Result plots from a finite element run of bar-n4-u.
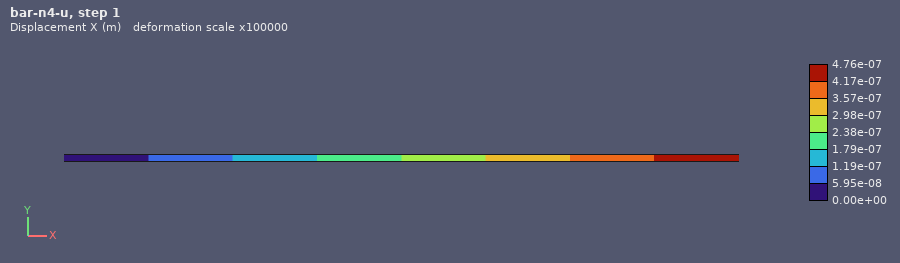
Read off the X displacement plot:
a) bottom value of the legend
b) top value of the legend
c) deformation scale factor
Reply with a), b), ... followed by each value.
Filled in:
a) 0.00e+00 m
b) 4.76e-07 m
c) 100000
